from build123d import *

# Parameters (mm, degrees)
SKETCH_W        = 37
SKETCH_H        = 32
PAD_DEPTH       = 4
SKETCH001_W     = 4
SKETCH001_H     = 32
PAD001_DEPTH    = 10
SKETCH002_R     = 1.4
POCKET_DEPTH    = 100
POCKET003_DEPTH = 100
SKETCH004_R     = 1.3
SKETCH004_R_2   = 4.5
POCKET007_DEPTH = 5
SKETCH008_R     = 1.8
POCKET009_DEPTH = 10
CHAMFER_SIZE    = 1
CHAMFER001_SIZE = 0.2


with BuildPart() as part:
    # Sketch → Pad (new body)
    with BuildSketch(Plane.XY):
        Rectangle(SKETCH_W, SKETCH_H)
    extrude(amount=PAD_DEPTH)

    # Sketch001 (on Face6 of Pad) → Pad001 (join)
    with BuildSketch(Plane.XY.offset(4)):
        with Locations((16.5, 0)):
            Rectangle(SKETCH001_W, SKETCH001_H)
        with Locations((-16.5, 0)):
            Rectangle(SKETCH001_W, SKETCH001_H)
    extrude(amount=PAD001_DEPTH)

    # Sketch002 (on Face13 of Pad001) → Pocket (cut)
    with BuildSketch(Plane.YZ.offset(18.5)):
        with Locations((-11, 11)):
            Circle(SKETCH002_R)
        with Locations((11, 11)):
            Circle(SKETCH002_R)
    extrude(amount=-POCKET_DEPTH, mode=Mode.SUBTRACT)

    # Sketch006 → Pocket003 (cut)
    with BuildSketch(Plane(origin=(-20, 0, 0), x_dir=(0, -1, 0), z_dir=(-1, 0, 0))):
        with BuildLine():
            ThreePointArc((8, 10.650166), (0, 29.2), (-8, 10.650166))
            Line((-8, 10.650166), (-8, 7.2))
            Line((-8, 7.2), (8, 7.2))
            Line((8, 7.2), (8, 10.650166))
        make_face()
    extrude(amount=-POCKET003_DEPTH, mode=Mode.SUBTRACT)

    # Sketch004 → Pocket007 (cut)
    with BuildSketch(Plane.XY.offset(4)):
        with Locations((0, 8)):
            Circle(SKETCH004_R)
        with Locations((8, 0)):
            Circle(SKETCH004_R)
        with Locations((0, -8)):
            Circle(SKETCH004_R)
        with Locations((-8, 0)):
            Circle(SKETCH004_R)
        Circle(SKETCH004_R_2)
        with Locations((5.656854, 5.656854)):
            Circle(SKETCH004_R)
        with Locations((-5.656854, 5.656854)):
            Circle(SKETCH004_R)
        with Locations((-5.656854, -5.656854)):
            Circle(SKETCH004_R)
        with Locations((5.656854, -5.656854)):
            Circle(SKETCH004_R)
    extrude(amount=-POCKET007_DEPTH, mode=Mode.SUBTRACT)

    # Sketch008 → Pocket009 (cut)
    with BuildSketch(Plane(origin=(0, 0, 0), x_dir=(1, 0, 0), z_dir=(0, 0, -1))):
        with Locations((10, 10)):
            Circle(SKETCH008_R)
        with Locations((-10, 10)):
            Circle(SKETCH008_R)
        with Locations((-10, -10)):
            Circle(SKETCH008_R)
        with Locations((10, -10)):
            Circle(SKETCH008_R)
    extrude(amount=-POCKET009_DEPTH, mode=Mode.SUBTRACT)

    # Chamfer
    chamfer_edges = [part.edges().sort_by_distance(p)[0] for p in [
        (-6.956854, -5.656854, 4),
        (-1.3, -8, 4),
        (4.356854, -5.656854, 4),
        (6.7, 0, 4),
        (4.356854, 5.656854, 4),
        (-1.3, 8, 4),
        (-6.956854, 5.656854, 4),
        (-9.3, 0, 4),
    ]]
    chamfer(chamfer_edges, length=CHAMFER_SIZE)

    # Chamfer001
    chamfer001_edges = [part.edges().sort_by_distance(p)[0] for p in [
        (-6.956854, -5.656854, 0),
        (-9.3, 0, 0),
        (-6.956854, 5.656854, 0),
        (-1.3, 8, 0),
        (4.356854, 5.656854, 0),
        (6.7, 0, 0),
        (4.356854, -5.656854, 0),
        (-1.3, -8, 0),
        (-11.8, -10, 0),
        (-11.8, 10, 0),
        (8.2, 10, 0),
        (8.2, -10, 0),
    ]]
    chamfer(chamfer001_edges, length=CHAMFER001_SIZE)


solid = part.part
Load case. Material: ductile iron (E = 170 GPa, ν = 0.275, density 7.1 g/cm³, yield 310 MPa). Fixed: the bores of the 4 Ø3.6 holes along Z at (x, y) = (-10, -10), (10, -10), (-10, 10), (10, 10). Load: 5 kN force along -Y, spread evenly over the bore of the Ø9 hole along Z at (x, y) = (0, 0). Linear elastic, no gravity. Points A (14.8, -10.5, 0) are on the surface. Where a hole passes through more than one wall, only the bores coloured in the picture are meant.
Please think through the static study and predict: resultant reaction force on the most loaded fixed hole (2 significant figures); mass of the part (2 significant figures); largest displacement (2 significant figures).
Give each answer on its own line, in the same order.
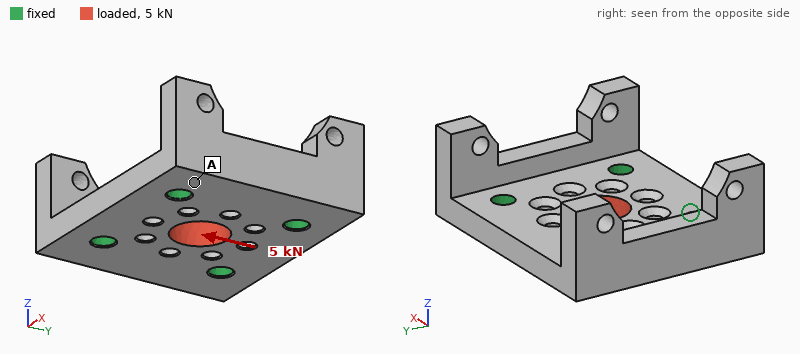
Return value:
1.3 kN
40 g
4.4 µm
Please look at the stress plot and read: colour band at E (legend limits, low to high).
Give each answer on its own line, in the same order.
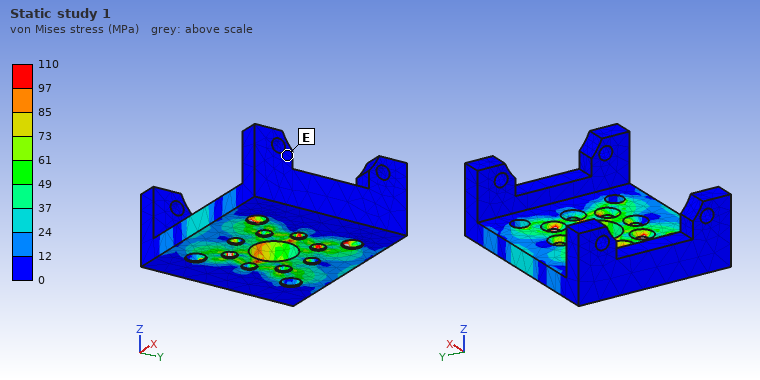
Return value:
0 to 12 MPa
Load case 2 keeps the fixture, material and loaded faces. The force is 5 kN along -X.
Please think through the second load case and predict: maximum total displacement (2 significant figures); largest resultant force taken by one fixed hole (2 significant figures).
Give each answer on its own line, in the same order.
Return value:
4.1 µm
1.3 kN
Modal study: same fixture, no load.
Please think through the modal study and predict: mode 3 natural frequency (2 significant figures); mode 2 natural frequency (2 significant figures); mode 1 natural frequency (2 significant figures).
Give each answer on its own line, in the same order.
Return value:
18 kHz
16 kHz
16 kHz
